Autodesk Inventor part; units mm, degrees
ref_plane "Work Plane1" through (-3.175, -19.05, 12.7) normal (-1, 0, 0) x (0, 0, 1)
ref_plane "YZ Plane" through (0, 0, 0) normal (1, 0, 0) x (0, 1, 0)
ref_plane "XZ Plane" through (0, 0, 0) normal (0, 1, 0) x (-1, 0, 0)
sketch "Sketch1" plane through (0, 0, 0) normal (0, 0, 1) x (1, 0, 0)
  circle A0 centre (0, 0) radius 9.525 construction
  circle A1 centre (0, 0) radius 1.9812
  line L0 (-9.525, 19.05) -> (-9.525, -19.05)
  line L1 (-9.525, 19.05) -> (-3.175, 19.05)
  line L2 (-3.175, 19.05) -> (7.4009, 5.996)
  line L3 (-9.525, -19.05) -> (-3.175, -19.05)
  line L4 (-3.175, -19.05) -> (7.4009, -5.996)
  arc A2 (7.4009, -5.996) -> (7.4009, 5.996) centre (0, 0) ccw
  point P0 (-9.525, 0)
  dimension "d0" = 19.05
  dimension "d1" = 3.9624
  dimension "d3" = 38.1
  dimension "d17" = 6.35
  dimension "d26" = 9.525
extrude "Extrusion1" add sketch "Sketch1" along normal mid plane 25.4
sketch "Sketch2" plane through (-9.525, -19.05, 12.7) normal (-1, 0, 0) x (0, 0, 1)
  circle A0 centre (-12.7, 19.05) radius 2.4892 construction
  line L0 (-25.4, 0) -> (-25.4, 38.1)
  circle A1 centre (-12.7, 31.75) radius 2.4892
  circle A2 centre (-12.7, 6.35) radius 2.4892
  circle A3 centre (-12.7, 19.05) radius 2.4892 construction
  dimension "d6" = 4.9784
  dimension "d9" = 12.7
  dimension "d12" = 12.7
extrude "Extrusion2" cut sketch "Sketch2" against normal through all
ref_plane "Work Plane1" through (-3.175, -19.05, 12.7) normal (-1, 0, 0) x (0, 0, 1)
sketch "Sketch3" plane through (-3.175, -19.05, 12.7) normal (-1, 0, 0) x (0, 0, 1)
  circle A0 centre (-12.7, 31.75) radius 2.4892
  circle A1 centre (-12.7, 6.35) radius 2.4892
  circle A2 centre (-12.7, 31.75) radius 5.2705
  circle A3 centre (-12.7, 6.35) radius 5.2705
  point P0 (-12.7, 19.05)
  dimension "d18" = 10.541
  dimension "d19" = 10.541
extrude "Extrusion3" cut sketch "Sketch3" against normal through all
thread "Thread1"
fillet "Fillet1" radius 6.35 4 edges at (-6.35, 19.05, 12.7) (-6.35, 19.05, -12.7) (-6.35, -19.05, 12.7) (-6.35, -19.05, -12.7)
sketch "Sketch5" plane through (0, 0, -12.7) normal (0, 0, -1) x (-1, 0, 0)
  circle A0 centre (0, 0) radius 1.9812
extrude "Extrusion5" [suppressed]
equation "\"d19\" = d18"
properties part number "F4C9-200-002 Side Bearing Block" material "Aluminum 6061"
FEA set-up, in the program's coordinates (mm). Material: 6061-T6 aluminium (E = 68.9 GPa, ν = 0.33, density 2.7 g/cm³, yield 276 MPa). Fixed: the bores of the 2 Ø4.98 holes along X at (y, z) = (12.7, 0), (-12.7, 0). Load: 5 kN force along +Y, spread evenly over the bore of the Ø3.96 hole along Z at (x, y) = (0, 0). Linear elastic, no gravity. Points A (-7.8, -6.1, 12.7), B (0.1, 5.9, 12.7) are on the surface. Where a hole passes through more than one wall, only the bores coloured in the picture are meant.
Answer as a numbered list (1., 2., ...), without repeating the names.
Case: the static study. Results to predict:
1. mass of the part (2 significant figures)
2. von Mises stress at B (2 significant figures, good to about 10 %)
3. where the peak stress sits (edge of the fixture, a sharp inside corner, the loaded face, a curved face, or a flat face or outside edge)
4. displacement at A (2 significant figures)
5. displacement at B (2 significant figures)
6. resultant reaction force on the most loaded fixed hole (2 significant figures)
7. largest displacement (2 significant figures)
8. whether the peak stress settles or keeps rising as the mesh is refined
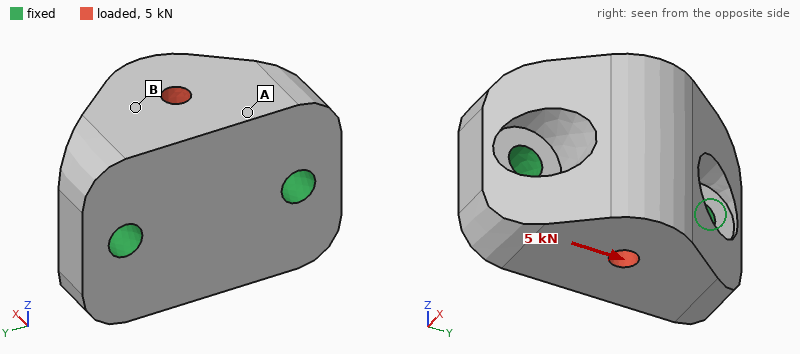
1. 31 g
2. 12 MPa
3. edge of the fixture
4. 2.9 µm
5. 5.0 µm
6. 2.8 kN
7. 7.0 µm
8. keeps rising
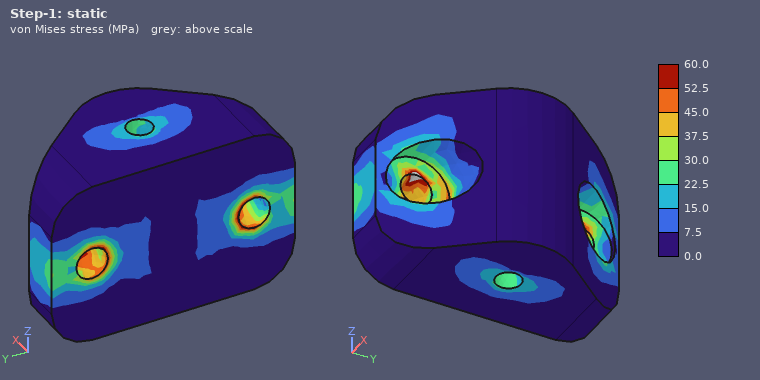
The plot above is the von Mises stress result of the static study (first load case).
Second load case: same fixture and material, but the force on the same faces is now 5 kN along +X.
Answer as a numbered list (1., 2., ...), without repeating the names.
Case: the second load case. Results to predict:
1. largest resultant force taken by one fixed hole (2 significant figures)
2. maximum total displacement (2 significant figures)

1. 2.6 kN
2. 10 µm
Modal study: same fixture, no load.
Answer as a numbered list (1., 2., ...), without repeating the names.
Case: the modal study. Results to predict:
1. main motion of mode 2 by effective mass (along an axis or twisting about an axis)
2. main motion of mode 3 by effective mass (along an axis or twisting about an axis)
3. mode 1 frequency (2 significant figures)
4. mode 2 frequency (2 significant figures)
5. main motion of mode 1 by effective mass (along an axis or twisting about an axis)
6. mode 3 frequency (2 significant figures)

1. along X
2. along Y
3. 13 kHz
4. 27 kHz
5. along Z
6. 29 kHz
